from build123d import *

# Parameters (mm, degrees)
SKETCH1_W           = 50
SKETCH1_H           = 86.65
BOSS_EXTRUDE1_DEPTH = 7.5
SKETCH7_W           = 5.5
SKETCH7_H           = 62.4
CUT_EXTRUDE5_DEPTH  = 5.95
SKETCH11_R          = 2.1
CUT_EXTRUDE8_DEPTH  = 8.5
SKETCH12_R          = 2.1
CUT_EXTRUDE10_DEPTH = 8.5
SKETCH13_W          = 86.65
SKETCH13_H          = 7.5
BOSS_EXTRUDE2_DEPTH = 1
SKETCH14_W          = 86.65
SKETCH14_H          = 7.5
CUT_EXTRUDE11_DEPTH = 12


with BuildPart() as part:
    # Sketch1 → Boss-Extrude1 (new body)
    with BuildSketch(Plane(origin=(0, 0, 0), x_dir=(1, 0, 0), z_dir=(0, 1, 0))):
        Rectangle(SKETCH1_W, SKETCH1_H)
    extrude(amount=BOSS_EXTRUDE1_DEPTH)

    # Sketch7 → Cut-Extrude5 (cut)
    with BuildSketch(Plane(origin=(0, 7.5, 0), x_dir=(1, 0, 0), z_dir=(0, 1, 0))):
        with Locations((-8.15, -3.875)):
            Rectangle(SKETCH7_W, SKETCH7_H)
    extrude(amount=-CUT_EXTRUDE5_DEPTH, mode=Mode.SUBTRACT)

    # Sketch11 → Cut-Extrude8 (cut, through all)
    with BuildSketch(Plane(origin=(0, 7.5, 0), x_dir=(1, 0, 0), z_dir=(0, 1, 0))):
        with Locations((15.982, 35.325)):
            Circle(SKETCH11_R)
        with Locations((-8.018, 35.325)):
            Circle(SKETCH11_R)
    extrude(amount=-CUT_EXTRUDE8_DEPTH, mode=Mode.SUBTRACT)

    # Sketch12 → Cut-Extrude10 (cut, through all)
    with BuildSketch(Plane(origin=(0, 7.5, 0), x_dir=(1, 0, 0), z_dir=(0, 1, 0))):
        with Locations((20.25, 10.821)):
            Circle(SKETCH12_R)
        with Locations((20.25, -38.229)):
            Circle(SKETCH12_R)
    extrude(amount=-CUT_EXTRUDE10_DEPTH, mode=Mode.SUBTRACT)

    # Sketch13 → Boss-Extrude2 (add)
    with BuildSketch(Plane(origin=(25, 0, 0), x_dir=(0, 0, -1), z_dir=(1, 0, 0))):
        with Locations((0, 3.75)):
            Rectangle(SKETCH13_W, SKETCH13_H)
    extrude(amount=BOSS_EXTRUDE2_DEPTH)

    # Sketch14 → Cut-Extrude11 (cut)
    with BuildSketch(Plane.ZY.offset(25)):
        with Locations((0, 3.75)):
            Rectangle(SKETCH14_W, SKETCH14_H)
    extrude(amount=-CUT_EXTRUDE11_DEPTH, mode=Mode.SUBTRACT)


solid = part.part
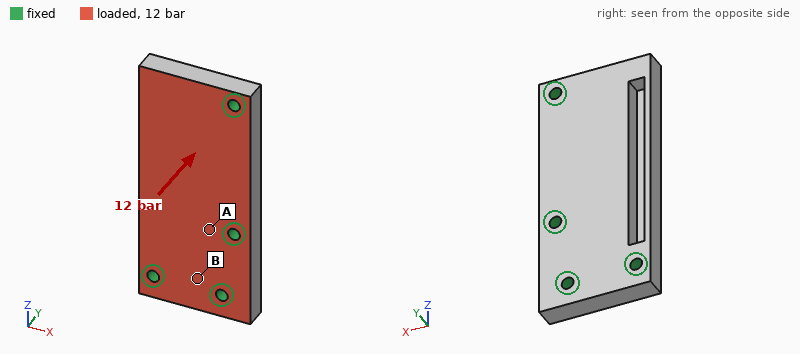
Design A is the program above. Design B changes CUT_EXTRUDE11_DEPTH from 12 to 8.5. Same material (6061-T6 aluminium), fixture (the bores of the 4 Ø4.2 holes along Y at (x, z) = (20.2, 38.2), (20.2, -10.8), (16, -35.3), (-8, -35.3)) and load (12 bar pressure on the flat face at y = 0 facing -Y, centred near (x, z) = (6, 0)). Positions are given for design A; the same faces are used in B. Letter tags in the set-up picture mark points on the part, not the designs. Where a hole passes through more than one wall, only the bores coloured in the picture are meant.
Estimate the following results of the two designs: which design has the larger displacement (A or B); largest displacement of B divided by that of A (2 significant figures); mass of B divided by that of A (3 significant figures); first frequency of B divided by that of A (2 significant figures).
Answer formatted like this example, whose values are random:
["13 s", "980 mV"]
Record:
["B", "1.3", "1.10", "0.83"]
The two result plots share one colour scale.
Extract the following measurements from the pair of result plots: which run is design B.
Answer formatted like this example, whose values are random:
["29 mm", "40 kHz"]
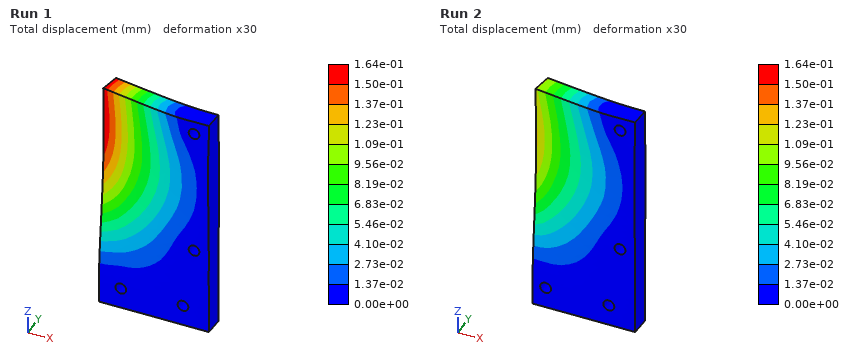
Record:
["Run 1"]
